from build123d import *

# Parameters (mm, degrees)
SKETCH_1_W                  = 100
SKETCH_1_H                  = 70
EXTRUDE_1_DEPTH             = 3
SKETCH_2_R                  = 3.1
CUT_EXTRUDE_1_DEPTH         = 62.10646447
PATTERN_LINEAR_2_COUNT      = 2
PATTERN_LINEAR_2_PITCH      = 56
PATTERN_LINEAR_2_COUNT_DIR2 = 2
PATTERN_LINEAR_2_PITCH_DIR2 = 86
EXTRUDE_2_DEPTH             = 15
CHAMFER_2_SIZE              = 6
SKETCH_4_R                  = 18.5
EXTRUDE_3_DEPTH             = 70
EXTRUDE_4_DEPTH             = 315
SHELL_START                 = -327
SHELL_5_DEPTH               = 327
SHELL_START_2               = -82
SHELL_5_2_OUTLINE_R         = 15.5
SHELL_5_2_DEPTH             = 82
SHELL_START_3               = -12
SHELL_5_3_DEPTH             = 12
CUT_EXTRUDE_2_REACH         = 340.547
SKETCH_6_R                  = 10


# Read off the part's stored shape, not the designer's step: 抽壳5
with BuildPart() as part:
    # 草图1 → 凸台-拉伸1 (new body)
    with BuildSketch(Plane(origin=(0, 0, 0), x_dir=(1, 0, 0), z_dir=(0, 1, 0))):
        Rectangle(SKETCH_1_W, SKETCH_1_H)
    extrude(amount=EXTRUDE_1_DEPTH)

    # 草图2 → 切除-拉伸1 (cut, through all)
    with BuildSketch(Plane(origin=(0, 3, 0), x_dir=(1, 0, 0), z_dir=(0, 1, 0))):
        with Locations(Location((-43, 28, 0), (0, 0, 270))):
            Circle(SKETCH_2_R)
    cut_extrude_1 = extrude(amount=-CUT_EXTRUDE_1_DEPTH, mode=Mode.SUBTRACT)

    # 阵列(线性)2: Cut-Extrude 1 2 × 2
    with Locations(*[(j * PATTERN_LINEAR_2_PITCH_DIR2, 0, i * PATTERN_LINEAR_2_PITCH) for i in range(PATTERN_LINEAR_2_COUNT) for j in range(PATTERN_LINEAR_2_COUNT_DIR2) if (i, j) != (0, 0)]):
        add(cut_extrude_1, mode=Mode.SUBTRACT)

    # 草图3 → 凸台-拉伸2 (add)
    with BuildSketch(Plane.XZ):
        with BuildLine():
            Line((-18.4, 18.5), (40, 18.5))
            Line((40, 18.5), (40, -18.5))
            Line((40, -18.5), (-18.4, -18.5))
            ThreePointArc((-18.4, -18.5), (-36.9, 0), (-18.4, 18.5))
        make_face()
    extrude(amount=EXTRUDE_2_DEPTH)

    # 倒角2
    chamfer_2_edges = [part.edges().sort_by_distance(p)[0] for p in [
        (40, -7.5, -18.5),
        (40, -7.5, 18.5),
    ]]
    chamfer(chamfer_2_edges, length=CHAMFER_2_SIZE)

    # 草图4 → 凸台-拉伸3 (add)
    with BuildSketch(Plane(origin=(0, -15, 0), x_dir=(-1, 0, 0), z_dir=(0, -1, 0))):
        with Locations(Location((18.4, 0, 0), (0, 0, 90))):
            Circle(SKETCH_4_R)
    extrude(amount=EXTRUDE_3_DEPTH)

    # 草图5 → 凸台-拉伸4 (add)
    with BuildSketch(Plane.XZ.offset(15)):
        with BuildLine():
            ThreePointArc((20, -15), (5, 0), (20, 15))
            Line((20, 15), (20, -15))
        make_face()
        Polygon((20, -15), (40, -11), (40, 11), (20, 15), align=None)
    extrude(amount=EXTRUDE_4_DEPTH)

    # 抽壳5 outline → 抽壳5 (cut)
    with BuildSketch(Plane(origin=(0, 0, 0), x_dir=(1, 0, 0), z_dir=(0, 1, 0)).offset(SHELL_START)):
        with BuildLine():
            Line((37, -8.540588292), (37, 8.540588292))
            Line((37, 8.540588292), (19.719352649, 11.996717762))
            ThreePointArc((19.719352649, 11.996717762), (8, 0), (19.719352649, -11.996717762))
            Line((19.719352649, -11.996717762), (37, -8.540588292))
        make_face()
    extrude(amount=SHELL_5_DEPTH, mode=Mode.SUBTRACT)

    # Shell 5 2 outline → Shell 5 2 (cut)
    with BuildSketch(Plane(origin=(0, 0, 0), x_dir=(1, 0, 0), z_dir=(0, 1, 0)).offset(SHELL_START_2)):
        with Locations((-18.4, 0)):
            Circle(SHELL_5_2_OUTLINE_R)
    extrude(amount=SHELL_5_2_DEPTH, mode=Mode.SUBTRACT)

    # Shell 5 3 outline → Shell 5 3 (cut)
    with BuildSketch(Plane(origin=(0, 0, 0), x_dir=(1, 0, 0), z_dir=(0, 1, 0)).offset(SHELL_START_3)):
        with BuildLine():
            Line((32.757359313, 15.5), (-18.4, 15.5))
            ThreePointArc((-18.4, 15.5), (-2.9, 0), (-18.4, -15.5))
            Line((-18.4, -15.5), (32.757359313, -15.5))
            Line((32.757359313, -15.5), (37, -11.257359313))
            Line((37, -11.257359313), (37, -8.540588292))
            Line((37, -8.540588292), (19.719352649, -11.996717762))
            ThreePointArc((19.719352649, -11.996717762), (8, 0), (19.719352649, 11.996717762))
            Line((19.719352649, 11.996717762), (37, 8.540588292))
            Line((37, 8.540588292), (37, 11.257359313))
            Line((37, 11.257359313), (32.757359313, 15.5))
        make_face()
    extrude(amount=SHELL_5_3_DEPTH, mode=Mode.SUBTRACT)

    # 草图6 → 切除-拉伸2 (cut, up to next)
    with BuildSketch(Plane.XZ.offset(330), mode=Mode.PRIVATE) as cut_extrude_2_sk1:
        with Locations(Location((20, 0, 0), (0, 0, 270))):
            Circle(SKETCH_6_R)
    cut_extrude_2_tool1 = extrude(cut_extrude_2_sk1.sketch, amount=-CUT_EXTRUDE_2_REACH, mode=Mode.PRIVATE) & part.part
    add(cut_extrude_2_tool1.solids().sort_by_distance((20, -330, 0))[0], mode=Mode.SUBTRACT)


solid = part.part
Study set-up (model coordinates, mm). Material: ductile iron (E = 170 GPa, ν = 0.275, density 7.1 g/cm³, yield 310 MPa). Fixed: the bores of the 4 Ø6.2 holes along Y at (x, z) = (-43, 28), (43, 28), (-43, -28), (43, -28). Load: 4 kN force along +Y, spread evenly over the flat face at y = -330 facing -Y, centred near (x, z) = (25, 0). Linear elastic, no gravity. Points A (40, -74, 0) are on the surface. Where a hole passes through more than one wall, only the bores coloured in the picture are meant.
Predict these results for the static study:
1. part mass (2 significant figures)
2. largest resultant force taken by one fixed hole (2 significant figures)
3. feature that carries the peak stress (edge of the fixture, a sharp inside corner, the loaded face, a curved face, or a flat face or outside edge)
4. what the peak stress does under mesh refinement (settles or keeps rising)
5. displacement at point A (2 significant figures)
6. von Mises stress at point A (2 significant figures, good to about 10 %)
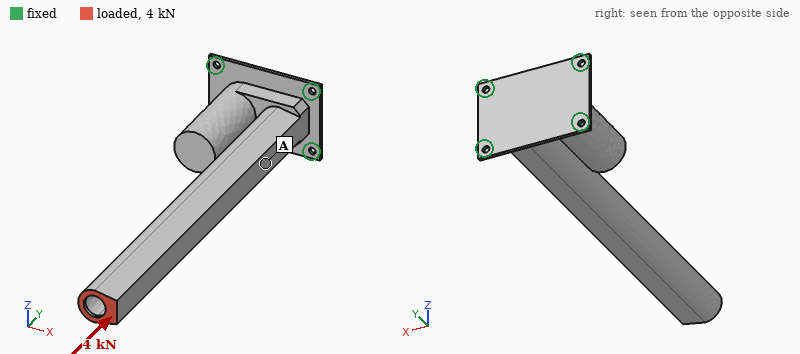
1.1 kg
1.8 kN
edge of the fixture
keeps rising
62 µm
16 MPa
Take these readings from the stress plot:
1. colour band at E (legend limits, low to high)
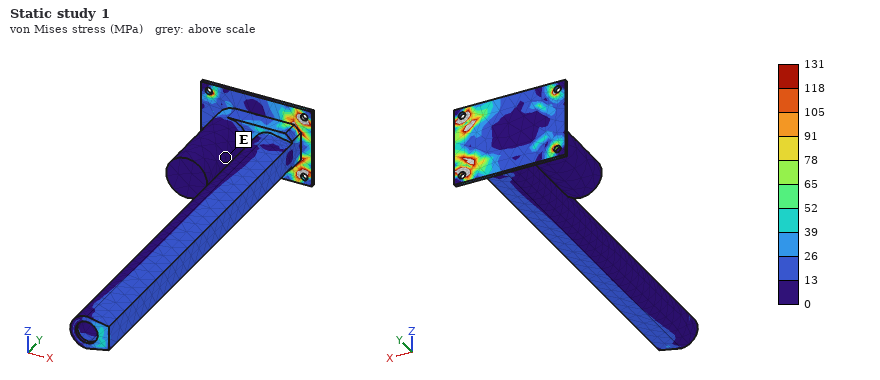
0 to 13 MPa
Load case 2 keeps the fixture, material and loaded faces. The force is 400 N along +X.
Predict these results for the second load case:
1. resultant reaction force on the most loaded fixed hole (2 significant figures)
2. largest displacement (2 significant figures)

1.2 kN
1.5 mm
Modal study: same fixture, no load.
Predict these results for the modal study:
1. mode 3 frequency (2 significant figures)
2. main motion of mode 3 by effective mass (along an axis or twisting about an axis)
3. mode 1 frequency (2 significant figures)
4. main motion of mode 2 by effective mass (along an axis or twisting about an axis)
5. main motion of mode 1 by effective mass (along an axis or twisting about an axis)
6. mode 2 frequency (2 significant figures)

1000 Hz
along Z
150 Hz
along X
along Z
180 Hz
